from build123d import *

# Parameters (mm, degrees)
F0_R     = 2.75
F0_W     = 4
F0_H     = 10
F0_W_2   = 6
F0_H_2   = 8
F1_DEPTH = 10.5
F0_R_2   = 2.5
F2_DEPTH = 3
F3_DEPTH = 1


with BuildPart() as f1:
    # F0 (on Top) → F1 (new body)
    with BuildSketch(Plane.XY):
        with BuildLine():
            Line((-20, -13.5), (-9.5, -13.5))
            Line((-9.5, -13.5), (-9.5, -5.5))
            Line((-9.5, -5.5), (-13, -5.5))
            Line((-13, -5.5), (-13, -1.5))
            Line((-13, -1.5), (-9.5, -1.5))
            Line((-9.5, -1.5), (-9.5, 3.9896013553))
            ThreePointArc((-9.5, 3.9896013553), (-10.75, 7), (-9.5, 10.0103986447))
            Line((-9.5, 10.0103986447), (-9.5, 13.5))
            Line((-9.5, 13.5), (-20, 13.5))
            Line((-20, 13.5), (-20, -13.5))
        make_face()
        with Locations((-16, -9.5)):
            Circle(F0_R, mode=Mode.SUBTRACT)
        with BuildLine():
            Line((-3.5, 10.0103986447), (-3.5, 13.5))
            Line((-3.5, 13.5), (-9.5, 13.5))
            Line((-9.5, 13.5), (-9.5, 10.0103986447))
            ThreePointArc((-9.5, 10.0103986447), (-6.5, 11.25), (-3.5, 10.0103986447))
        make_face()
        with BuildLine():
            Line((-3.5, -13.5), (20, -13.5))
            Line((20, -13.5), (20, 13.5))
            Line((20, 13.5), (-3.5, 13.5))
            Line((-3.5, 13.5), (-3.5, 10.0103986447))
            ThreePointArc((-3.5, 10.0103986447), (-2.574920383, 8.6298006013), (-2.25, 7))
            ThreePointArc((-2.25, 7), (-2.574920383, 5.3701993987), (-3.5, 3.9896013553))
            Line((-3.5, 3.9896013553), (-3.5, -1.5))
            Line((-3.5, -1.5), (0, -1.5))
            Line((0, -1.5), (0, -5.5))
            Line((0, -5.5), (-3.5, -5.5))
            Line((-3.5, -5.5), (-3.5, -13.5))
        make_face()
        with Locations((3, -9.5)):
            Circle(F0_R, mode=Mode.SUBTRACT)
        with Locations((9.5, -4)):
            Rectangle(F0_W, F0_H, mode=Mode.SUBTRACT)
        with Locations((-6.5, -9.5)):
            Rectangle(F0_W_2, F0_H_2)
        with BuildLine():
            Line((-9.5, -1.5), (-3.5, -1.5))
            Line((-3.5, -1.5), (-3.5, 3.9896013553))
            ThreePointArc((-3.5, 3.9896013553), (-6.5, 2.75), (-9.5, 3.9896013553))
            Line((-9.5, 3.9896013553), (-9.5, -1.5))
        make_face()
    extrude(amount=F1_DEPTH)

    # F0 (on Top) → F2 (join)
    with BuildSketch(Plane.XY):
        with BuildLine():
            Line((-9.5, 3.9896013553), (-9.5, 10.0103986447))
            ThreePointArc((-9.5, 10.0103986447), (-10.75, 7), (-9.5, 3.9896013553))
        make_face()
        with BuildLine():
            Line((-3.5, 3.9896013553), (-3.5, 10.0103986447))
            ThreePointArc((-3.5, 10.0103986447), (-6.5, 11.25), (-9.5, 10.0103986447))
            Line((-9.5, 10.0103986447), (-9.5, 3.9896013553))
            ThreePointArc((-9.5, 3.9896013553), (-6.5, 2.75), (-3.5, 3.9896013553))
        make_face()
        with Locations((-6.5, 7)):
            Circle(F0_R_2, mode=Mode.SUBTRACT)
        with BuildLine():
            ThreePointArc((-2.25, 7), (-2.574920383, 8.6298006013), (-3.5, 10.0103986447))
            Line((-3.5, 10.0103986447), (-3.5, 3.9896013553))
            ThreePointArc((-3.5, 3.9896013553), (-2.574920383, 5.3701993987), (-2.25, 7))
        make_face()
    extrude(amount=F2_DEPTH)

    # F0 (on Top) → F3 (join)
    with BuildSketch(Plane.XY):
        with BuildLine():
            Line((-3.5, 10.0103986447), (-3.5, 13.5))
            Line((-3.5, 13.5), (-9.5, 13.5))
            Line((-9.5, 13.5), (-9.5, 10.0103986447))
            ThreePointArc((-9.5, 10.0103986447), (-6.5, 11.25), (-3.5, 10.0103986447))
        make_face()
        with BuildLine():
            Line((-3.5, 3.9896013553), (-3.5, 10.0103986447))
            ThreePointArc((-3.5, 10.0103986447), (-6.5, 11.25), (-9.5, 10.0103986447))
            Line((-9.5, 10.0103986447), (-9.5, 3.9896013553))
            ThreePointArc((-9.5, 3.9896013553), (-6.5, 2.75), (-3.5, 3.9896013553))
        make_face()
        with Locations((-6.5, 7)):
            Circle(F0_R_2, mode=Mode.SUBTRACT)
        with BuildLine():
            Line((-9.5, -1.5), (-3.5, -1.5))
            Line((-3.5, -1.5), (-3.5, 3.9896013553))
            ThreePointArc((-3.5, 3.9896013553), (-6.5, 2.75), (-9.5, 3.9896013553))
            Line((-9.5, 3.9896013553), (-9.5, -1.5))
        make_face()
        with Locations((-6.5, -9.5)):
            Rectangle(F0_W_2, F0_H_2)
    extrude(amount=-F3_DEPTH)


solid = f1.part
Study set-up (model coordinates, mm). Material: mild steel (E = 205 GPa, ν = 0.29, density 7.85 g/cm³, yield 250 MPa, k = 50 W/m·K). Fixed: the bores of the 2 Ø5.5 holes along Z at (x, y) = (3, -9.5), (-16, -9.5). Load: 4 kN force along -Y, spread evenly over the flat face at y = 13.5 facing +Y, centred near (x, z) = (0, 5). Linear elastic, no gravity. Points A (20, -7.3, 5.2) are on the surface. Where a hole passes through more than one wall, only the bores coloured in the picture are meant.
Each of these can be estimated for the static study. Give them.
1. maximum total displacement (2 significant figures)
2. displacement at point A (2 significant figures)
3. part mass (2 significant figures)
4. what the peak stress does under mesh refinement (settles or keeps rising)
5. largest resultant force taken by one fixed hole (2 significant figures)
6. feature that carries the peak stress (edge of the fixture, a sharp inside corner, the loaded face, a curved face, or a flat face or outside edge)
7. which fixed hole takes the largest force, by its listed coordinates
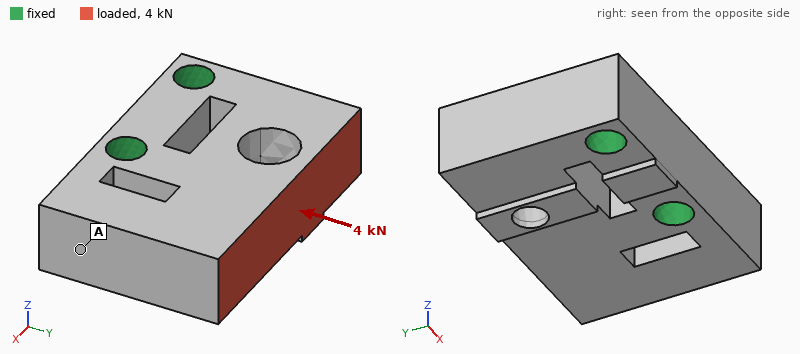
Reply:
5.7 µm
4.1 µm
75 g
keeps rising
3.0 kN
edge of the fixture
(3, -9.5)
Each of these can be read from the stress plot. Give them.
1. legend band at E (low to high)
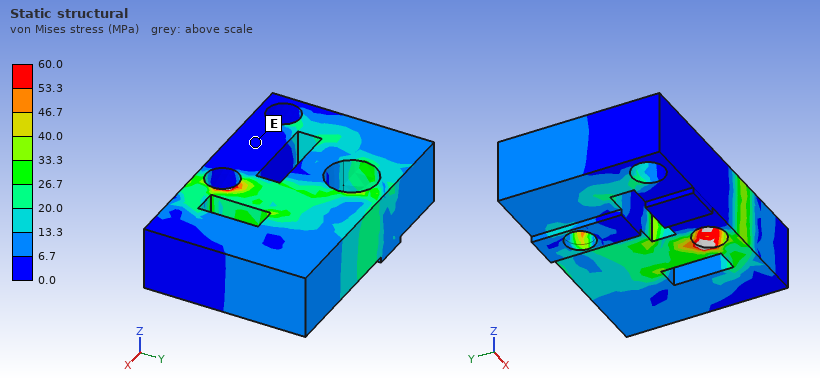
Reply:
0.0 to 6.7 MPa
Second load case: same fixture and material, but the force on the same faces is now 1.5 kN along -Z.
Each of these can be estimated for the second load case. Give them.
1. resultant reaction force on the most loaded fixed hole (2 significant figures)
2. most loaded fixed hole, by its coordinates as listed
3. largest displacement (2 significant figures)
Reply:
1.1 kN
(3, -9.5)
21 µm
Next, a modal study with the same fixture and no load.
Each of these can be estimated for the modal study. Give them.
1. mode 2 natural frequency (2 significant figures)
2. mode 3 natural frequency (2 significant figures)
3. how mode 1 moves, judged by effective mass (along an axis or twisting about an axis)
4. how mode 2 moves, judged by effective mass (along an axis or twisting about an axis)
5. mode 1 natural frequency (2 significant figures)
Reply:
14 kHz
16 kHz
along Z
along X
9800 Hz
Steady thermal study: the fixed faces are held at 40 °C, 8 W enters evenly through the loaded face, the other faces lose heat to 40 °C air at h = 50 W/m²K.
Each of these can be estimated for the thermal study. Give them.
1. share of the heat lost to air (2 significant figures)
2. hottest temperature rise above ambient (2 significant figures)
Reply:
13 %
13 K
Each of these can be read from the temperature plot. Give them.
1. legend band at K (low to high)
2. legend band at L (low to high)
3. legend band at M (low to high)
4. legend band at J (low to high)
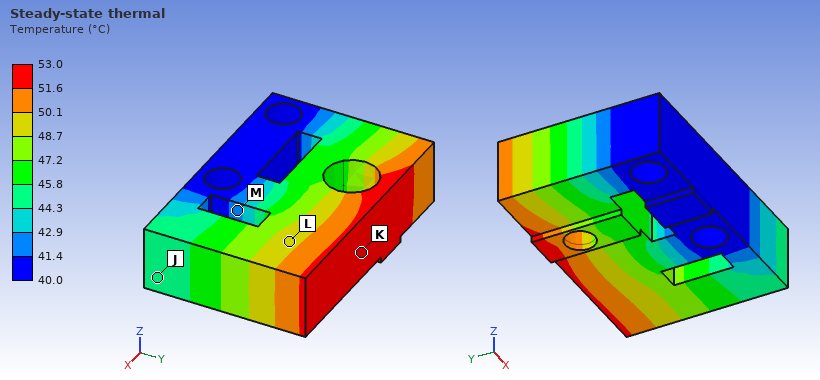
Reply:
51.6 to 53.0 °C
48.7 to 50.1 °C
41.4 to 42.9 °C
44.3 to 45.8 °C
